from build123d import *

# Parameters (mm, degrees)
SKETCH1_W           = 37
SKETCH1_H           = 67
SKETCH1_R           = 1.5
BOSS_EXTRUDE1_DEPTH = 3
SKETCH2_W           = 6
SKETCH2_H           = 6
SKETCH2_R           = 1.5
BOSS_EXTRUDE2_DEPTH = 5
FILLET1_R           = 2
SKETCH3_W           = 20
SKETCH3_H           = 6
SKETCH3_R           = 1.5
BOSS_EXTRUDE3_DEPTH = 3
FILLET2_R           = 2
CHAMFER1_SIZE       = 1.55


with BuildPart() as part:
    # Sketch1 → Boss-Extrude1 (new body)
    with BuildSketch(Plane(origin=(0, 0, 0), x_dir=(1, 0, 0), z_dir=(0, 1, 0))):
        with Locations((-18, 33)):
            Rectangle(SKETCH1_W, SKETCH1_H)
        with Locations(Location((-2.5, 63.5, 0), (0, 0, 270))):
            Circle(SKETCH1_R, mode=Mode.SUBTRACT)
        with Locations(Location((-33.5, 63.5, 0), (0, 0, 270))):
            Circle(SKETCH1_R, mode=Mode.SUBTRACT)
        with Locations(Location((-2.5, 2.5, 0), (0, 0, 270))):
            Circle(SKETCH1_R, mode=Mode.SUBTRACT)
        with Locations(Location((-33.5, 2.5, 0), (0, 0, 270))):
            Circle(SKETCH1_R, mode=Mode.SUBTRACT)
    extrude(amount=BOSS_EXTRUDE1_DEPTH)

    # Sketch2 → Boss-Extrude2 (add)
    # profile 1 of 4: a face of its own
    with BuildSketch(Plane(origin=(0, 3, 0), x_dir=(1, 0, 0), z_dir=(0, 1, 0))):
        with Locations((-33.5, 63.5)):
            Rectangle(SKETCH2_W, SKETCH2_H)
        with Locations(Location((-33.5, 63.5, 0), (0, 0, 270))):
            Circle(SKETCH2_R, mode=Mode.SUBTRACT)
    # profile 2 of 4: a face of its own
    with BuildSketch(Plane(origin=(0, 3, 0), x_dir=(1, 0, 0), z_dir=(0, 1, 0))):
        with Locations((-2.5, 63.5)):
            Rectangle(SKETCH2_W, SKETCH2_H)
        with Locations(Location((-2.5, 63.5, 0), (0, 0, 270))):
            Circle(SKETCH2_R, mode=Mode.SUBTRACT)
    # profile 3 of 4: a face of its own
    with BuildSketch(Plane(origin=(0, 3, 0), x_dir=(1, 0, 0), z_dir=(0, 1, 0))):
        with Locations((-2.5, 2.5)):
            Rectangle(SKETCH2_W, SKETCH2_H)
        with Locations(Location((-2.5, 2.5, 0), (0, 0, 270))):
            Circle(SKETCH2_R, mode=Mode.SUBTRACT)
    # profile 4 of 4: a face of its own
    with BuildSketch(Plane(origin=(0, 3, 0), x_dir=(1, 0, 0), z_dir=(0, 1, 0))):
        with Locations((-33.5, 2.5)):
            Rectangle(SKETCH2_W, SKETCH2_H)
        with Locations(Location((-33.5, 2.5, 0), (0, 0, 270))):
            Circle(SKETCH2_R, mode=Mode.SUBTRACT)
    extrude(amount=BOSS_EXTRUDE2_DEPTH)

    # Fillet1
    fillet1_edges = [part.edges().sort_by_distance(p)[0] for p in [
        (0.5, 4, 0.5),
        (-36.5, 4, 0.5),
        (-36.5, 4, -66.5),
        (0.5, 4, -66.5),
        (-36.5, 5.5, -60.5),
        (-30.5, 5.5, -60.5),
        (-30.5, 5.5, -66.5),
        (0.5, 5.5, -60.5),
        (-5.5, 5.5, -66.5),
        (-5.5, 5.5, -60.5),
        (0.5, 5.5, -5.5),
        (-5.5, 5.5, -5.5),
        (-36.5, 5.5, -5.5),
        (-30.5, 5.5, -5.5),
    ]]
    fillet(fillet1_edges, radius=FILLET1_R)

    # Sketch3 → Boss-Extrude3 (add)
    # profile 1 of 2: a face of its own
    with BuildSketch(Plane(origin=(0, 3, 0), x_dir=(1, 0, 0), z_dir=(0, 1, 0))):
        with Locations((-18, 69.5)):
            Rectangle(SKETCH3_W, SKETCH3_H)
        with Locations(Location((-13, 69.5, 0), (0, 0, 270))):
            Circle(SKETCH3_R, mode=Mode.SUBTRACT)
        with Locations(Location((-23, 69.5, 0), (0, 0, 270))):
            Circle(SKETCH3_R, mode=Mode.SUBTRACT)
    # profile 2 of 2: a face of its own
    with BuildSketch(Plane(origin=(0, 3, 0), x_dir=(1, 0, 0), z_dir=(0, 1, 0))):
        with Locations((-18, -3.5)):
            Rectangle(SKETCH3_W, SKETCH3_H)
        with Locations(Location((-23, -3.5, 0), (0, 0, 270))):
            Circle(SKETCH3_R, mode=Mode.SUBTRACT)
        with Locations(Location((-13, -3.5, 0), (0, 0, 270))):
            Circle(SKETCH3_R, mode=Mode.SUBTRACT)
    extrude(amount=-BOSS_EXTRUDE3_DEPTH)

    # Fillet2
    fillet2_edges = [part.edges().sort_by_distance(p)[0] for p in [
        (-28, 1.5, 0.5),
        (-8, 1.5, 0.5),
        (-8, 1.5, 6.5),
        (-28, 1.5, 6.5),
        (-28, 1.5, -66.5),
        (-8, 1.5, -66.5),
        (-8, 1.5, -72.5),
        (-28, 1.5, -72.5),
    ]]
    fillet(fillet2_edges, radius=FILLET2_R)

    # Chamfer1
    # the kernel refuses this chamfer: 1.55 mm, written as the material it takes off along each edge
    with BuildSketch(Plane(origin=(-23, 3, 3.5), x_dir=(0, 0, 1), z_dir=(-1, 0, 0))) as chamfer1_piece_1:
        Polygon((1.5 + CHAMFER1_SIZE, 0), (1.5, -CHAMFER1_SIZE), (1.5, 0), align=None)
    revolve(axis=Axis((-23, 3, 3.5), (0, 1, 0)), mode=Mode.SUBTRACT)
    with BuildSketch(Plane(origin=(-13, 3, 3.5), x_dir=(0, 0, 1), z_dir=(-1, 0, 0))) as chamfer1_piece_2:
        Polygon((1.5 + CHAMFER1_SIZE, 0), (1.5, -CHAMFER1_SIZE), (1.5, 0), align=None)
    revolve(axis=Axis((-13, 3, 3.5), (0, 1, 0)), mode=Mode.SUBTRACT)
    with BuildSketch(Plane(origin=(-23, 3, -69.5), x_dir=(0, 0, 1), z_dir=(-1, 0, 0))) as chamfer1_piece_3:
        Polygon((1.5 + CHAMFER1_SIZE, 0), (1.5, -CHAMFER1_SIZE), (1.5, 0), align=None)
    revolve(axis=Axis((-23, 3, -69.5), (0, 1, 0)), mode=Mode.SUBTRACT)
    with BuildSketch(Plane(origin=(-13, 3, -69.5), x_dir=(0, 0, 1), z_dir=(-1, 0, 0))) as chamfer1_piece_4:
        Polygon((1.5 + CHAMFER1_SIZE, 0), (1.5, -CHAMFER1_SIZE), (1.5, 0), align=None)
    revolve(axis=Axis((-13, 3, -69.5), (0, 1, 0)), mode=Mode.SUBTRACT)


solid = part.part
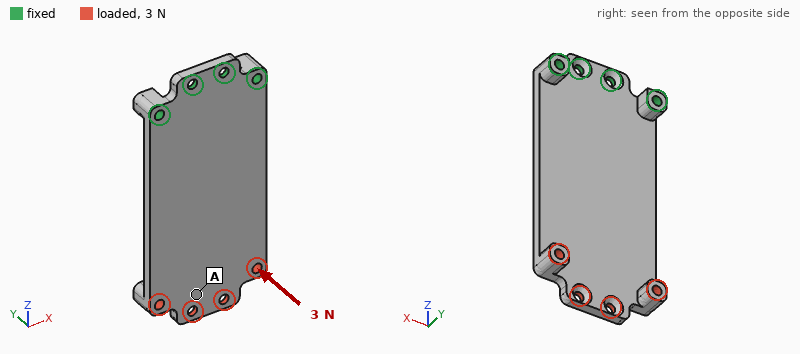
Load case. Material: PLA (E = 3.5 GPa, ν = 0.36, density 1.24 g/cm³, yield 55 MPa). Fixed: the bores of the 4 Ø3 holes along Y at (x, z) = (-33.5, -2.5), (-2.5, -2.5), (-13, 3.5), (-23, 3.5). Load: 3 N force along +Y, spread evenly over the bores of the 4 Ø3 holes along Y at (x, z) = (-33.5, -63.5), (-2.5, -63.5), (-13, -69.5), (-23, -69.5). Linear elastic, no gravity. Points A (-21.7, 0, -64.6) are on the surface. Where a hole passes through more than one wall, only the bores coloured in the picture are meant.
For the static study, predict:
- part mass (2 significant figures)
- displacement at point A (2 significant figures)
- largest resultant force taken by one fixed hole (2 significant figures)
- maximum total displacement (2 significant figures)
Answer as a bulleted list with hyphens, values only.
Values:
- 10 g
- 0.81 mm
- 5.1 N
- 0.96 mm
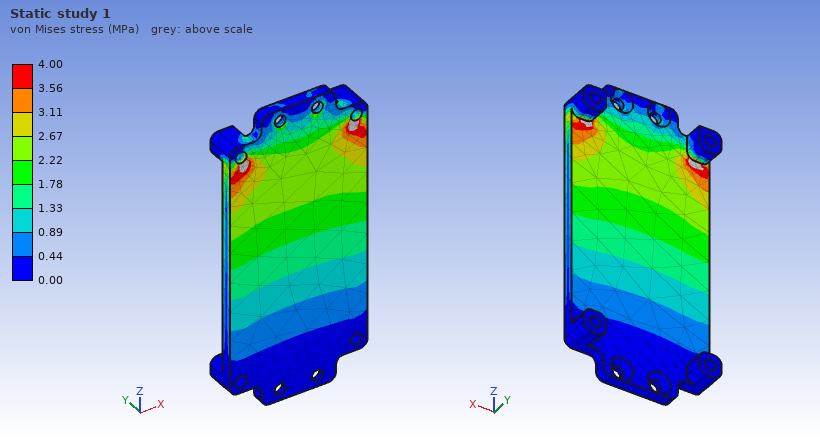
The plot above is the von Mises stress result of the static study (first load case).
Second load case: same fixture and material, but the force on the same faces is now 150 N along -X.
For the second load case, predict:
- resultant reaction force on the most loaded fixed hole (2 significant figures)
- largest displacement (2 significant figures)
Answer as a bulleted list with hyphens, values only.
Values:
- 290 N
- 0.93 mm
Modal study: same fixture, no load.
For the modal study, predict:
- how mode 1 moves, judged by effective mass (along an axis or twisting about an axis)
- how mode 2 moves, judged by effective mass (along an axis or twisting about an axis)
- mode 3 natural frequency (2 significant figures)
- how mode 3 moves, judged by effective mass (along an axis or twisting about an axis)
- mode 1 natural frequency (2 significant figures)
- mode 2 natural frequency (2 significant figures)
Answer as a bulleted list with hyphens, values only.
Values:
- along Y
- twisting about Z
- 1100 Hz
- along Y
- 180 Hz
- 690 Hz
